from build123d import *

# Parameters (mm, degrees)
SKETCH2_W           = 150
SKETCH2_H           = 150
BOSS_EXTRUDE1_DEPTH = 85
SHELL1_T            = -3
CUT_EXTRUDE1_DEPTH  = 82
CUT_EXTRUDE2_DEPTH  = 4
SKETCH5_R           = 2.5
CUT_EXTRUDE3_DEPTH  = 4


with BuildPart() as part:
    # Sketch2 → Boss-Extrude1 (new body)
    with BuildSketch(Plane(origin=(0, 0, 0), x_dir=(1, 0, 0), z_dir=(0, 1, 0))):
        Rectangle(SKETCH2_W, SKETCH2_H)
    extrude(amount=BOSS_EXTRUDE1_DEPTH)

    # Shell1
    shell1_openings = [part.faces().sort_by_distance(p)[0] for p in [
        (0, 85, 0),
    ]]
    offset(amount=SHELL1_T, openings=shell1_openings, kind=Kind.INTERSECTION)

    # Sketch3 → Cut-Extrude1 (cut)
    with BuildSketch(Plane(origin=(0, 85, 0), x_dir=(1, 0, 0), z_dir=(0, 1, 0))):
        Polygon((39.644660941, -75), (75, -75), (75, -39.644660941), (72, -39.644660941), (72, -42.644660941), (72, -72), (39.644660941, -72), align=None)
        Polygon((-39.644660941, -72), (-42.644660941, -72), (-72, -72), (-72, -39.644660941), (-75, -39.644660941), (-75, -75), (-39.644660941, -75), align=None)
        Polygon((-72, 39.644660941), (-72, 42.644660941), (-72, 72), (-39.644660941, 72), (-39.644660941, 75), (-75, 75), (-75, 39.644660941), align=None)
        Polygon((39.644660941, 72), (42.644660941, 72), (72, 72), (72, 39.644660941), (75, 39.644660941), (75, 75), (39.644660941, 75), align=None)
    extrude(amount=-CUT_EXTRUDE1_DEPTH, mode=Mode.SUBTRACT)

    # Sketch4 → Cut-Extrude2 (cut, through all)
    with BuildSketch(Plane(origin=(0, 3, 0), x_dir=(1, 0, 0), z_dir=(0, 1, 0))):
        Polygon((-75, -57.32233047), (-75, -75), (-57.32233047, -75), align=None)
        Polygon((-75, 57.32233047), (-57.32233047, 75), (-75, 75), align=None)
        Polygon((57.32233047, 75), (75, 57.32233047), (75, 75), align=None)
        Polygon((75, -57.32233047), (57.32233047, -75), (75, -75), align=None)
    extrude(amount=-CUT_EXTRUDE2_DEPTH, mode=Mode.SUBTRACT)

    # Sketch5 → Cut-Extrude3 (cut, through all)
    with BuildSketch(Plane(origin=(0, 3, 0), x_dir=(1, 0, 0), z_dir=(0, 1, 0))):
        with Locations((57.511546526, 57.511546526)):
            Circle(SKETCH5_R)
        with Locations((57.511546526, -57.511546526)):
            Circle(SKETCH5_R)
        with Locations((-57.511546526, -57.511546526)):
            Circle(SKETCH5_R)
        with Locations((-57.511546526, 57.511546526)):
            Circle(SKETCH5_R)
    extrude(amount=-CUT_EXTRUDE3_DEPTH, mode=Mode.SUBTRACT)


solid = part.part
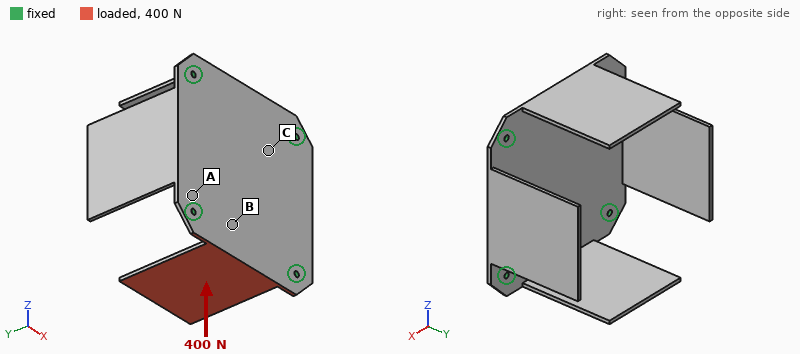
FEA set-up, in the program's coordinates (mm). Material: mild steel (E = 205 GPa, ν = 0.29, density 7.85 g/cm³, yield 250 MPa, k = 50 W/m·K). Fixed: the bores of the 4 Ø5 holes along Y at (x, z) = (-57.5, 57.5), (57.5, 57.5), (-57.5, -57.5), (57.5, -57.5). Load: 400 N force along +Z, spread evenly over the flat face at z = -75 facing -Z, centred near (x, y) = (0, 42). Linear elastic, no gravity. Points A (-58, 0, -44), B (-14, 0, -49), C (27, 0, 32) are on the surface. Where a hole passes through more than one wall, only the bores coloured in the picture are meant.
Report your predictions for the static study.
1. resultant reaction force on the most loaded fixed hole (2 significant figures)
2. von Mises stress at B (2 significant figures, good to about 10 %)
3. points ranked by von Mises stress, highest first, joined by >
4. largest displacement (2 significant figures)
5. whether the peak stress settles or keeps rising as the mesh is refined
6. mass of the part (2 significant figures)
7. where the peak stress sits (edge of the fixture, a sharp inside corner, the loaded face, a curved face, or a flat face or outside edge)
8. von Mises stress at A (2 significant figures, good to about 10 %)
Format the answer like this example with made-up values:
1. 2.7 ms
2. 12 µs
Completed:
1. 140 N
2. 47 MPa
3. B > A > C
4. 1.4 mm
5. keeps rising
6. 1.1 kg
7. edge of the fixture
8. 26 MPa
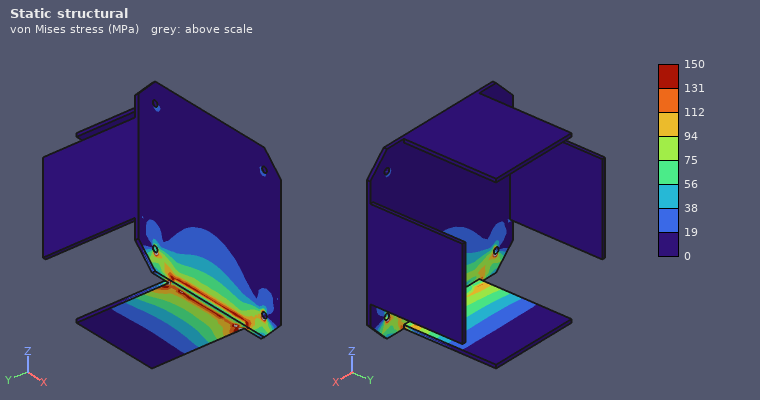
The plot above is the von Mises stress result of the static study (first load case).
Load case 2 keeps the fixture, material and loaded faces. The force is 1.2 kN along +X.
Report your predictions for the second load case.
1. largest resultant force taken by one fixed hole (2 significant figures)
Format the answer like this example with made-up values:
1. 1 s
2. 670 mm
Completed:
1. 800 N
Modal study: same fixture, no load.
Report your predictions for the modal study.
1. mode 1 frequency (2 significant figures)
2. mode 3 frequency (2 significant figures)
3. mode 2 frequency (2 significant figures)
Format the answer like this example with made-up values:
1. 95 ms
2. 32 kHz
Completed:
1. 250 Hz
2. 270 Hz
3. 270 Hz
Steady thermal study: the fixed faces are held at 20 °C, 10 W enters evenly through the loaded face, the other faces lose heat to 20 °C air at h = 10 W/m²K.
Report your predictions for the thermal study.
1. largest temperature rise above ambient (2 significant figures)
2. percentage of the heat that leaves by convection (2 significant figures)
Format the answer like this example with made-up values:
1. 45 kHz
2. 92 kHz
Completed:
1. 42 K
2. 49 %
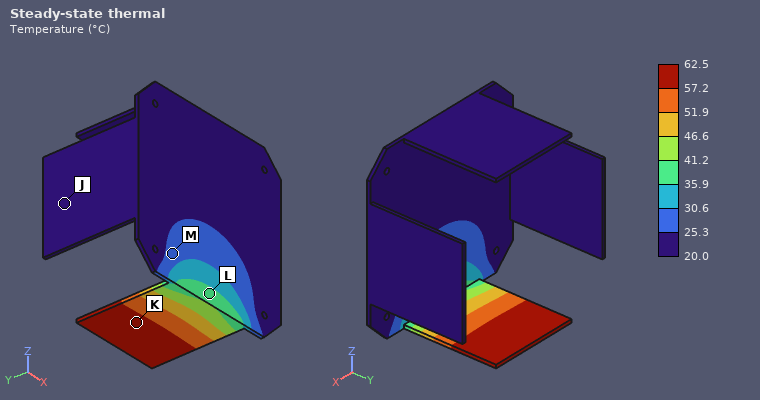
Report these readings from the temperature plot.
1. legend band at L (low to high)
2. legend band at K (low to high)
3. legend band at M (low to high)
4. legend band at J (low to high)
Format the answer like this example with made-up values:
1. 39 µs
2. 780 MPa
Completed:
1. 35.9 to 41.2 °C
2. 57.2 to 62.5 °C
3. 25.3 to 30.6 °C
4. 20.0 to 25.3 °C
